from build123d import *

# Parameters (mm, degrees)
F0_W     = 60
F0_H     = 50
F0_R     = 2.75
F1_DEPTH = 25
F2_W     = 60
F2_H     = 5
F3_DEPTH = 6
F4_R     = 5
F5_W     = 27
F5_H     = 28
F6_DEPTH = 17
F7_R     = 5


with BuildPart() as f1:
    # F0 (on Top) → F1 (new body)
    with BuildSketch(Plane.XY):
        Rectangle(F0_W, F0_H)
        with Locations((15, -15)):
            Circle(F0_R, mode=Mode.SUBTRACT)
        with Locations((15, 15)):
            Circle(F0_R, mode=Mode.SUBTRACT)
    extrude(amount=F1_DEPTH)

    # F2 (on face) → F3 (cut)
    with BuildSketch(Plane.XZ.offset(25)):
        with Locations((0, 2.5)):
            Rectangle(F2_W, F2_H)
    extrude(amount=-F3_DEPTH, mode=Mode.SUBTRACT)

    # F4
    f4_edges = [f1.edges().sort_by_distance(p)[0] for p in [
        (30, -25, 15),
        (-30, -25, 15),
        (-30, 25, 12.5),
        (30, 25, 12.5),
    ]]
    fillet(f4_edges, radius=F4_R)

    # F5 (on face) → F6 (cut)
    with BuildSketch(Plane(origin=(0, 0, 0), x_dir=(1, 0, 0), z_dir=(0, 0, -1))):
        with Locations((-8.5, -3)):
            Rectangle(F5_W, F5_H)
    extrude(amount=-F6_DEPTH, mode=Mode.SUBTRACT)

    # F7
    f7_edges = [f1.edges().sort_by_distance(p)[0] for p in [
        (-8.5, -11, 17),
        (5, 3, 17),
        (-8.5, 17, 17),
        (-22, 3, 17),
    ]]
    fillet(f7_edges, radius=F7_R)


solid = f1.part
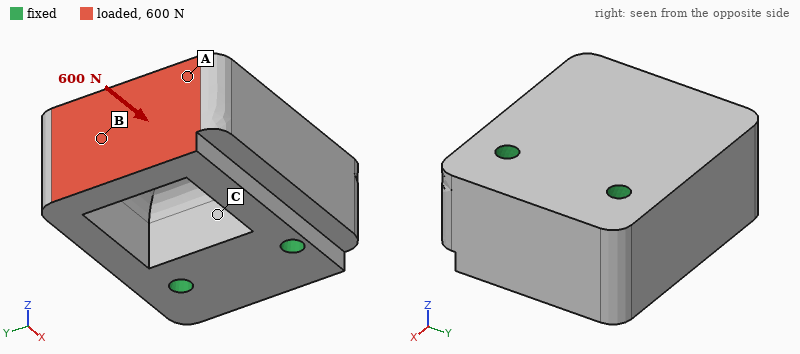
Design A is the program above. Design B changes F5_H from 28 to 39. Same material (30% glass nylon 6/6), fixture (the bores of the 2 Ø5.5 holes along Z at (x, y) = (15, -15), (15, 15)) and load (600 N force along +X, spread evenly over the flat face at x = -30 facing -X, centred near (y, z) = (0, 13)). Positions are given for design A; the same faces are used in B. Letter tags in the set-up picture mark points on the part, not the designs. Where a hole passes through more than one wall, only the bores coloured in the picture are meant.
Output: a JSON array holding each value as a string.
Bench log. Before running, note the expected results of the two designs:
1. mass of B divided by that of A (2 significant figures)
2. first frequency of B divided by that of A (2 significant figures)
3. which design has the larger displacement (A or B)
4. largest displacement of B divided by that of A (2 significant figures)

["0.92", "0.81", "B", "2.3"]
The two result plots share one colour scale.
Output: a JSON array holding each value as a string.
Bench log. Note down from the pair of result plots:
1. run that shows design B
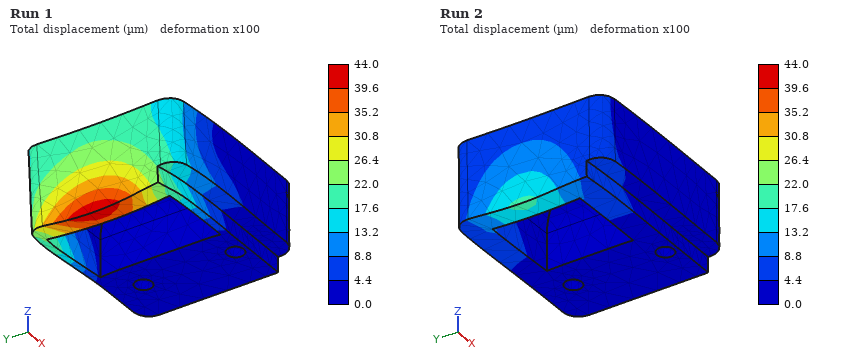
["Run 1"]
